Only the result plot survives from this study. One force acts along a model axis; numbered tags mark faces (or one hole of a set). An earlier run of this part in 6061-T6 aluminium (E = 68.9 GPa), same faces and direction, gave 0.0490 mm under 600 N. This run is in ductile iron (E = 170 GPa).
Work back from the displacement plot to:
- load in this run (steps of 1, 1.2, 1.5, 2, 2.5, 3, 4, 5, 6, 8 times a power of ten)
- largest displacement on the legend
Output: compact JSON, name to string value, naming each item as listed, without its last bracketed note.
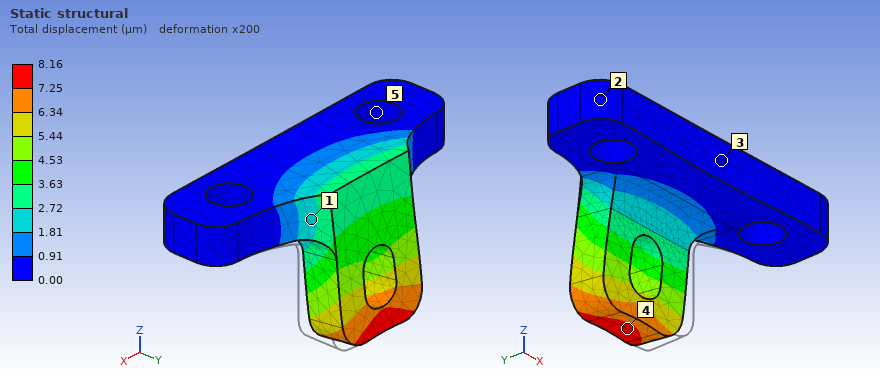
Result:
{"load in this run": "250 N", "largest displacement on the legend": "8.16 µm"}
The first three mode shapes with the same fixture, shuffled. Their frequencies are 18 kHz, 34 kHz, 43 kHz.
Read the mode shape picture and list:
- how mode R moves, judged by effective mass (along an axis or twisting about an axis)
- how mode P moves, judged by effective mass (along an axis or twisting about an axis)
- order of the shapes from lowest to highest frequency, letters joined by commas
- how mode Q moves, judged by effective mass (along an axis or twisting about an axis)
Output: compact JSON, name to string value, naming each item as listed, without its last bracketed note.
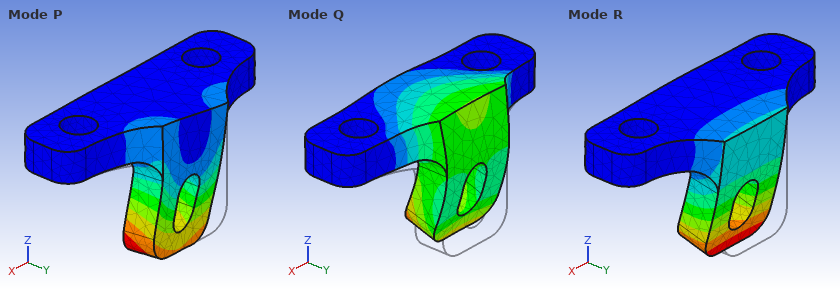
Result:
{"how mode R moves, judged by effective mass": "along Y", "how mode P moves, judged by effective mass": "along X", "order of the shapes from lowest to highest frequency, letters joined by commas": "R, P, Q", "how mode Q moves, judged by effective mass": "along Z"}
